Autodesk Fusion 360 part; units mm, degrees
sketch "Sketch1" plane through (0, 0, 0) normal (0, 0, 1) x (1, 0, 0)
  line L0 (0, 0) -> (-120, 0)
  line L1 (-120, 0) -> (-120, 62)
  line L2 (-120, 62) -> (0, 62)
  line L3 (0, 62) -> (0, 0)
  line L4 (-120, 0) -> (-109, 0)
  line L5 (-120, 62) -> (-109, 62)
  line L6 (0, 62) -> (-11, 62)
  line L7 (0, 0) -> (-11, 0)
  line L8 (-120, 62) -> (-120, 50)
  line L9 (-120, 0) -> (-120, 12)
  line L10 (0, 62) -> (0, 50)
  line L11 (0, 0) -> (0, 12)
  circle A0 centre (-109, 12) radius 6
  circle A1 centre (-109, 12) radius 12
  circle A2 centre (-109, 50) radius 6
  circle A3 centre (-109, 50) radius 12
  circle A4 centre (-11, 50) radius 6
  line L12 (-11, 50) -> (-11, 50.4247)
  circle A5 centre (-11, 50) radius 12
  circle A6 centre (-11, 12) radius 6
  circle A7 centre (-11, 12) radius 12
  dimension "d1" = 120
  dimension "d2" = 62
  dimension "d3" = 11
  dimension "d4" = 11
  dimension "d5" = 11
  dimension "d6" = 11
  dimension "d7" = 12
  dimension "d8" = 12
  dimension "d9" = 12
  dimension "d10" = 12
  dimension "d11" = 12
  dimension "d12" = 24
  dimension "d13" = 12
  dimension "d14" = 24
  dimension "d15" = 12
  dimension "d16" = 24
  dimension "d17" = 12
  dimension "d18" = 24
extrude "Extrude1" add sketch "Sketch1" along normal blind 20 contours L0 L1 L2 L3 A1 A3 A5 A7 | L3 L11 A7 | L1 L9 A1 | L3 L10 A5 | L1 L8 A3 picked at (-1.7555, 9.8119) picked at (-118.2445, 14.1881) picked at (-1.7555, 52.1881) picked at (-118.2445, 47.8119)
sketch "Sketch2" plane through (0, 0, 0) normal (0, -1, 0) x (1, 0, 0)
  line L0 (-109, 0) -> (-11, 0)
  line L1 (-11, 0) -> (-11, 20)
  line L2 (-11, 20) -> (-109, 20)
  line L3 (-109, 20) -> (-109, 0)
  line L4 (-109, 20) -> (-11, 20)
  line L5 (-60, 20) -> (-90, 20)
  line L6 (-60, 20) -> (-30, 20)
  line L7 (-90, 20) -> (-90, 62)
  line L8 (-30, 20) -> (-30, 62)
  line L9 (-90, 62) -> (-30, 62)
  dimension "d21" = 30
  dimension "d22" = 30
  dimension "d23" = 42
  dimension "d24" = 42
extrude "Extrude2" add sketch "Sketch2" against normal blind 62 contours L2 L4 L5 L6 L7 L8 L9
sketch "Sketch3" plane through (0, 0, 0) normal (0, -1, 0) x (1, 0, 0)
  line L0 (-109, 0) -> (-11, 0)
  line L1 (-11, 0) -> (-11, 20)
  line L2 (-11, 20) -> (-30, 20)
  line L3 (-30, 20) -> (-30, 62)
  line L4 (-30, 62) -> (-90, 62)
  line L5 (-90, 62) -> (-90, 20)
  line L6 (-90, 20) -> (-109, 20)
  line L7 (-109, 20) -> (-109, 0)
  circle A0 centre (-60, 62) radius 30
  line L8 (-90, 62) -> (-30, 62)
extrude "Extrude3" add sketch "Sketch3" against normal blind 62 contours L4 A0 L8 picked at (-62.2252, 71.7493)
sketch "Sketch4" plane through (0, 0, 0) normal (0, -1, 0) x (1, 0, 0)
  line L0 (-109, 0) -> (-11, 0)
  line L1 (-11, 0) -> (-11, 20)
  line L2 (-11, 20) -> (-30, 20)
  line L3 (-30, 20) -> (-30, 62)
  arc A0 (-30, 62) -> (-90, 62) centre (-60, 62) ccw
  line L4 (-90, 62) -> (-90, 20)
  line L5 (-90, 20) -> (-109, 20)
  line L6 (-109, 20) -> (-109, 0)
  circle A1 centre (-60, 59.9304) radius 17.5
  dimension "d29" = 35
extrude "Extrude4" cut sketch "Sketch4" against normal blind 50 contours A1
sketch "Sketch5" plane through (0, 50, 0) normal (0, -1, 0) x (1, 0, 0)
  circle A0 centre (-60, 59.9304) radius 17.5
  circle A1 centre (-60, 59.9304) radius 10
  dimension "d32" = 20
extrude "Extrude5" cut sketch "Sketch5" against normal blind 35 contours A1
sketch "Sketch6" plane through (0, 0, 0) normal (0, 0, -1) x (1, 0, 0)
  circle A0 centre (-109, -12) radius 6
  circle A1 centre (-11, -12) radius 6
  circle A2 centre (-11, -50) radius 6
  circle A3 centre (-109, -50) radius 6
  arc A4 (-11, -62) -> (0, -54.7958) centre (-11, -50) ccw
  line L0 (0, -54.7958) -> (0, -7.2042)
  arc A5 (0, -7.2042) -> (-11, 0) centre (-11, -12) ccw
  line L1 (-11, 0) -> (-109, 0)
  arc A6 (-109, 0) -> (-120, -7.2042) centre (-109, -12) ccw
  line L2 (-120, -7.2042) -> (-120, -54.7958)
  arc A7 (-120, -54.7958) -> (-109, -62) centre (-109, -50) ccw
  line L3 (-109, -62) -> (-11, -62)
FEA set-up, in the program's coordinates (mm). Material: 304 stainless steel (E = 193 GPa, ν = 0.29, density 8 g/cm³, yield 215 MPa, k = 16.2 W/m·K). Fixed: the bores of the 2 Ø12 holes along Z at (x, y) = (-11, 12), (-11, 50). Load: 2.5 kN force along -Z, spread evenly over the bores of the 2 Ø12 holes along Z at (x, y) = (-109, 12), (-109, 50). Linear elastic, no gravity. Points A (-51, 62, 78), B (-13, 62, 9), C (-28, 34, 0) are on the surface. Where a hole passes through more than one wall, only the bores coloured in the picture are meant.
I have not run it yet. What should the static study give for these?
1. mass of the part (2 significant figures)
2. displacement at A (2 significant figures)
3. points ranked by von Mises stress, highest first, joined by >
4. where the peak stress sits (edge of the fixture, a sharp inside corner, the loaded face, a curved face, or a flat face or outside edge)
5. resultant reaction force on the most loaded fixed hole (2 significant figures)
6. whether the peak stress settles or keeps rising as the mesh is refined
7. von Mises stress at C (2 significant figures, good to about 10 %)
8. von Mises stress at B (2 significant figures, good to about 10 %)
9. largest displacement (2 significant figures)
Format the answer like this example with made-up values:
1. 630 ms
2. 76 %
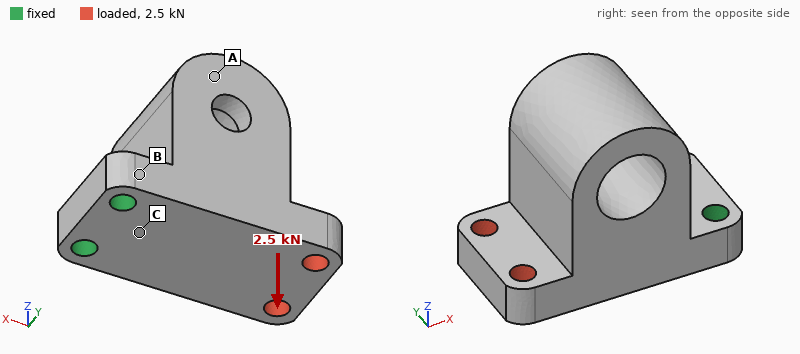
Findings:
1. 2.6 kg
2. 52 µm
3. C > B > A
4. edge of the fixture
5. 1.3 kN
6. keeps rising
7. 37 MPa
8. 17 MPa
9. 75 µm
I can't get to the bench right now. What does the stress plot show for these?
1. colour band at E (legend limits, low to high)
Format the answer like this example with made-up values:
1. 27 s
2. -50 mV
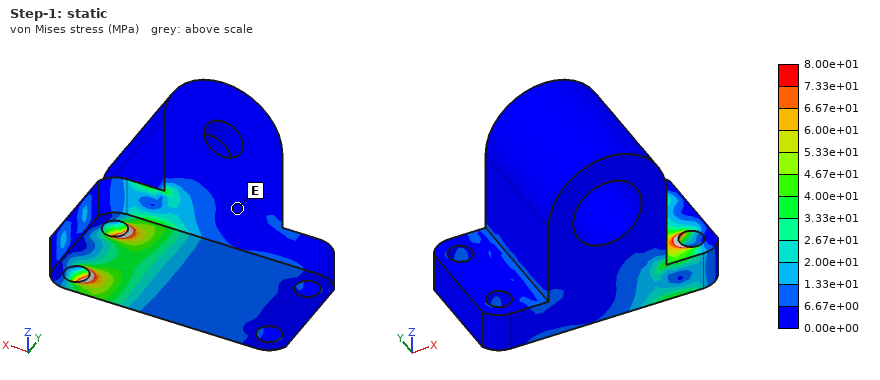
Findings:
1. 0.00e+00 to 6.67e+00 MPa
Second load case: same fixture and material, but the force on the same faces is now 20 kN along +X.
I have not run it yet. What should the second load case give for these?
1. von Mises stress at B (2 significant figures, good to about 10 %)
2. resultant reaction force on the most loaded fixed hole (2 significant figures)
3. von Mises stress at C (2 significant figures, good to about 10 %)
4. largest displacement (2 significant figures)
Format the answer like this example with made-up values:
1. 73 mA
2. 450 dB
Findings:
1. 9.0 MPa
2. 10 kN
3. 12 MPa
4. 15 µm
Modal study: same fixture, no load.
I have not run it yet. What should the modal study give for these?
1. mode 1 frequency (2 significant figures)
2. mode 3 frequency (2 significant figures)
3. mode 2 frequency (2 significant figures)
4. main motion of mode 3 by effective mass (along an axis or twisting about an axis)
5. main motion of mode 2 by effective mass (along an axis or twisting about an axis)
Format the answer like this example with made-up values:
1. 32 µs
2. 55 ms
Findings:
1. 940 Hz
2. 3300 Hz
3. 2100 Hz
4. along Y
5. along Y
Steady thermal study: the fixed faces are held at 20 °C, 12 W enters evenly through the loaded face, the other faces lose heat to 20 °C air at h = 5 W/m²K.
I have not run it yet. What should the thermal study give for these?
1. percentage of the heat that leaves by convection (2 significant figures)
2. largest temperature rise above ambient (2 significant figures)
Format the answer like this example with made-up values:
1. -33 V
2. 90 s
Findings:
1. 28 %
2. 42 K
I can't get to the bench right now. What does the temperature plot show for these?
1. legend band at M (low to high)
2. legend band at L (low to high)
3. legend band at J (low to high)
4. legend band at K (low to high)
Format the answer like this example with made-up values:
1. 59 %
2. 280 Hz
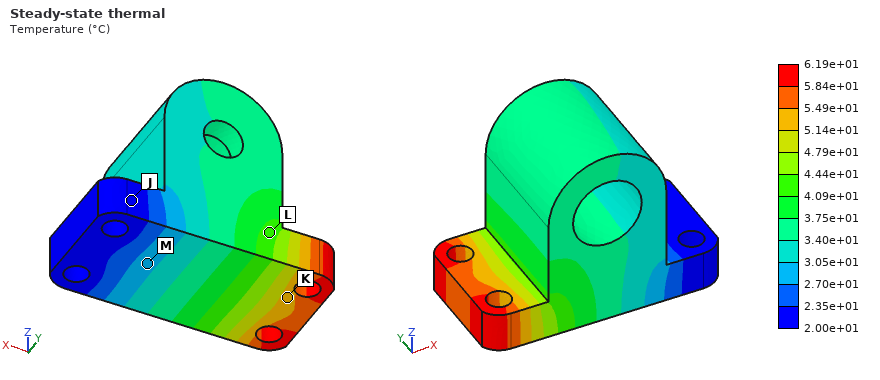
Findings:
1. 2.70e+01 to 3.05e+01 °C
2. 4.09e+01 to 4.44e+01 °C
3. 2.00e+01 to 2.35e+01 °C
4. 5.14e+01 to 5.49e+01 °C
